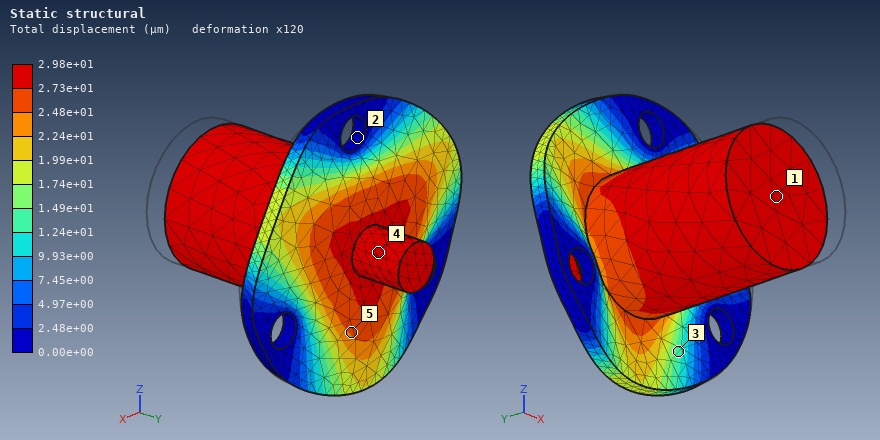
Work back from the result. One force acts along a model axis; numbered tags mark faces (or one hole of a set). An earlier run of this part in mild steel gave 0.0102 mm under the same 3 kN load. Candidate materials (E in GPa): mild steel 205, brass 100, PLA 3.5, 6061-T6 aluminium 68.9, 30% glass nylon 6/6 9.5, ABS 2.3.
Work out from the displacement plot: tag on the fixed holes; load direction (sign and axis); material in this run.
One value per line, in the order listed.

2
+Y
6061-T6 aluminium
